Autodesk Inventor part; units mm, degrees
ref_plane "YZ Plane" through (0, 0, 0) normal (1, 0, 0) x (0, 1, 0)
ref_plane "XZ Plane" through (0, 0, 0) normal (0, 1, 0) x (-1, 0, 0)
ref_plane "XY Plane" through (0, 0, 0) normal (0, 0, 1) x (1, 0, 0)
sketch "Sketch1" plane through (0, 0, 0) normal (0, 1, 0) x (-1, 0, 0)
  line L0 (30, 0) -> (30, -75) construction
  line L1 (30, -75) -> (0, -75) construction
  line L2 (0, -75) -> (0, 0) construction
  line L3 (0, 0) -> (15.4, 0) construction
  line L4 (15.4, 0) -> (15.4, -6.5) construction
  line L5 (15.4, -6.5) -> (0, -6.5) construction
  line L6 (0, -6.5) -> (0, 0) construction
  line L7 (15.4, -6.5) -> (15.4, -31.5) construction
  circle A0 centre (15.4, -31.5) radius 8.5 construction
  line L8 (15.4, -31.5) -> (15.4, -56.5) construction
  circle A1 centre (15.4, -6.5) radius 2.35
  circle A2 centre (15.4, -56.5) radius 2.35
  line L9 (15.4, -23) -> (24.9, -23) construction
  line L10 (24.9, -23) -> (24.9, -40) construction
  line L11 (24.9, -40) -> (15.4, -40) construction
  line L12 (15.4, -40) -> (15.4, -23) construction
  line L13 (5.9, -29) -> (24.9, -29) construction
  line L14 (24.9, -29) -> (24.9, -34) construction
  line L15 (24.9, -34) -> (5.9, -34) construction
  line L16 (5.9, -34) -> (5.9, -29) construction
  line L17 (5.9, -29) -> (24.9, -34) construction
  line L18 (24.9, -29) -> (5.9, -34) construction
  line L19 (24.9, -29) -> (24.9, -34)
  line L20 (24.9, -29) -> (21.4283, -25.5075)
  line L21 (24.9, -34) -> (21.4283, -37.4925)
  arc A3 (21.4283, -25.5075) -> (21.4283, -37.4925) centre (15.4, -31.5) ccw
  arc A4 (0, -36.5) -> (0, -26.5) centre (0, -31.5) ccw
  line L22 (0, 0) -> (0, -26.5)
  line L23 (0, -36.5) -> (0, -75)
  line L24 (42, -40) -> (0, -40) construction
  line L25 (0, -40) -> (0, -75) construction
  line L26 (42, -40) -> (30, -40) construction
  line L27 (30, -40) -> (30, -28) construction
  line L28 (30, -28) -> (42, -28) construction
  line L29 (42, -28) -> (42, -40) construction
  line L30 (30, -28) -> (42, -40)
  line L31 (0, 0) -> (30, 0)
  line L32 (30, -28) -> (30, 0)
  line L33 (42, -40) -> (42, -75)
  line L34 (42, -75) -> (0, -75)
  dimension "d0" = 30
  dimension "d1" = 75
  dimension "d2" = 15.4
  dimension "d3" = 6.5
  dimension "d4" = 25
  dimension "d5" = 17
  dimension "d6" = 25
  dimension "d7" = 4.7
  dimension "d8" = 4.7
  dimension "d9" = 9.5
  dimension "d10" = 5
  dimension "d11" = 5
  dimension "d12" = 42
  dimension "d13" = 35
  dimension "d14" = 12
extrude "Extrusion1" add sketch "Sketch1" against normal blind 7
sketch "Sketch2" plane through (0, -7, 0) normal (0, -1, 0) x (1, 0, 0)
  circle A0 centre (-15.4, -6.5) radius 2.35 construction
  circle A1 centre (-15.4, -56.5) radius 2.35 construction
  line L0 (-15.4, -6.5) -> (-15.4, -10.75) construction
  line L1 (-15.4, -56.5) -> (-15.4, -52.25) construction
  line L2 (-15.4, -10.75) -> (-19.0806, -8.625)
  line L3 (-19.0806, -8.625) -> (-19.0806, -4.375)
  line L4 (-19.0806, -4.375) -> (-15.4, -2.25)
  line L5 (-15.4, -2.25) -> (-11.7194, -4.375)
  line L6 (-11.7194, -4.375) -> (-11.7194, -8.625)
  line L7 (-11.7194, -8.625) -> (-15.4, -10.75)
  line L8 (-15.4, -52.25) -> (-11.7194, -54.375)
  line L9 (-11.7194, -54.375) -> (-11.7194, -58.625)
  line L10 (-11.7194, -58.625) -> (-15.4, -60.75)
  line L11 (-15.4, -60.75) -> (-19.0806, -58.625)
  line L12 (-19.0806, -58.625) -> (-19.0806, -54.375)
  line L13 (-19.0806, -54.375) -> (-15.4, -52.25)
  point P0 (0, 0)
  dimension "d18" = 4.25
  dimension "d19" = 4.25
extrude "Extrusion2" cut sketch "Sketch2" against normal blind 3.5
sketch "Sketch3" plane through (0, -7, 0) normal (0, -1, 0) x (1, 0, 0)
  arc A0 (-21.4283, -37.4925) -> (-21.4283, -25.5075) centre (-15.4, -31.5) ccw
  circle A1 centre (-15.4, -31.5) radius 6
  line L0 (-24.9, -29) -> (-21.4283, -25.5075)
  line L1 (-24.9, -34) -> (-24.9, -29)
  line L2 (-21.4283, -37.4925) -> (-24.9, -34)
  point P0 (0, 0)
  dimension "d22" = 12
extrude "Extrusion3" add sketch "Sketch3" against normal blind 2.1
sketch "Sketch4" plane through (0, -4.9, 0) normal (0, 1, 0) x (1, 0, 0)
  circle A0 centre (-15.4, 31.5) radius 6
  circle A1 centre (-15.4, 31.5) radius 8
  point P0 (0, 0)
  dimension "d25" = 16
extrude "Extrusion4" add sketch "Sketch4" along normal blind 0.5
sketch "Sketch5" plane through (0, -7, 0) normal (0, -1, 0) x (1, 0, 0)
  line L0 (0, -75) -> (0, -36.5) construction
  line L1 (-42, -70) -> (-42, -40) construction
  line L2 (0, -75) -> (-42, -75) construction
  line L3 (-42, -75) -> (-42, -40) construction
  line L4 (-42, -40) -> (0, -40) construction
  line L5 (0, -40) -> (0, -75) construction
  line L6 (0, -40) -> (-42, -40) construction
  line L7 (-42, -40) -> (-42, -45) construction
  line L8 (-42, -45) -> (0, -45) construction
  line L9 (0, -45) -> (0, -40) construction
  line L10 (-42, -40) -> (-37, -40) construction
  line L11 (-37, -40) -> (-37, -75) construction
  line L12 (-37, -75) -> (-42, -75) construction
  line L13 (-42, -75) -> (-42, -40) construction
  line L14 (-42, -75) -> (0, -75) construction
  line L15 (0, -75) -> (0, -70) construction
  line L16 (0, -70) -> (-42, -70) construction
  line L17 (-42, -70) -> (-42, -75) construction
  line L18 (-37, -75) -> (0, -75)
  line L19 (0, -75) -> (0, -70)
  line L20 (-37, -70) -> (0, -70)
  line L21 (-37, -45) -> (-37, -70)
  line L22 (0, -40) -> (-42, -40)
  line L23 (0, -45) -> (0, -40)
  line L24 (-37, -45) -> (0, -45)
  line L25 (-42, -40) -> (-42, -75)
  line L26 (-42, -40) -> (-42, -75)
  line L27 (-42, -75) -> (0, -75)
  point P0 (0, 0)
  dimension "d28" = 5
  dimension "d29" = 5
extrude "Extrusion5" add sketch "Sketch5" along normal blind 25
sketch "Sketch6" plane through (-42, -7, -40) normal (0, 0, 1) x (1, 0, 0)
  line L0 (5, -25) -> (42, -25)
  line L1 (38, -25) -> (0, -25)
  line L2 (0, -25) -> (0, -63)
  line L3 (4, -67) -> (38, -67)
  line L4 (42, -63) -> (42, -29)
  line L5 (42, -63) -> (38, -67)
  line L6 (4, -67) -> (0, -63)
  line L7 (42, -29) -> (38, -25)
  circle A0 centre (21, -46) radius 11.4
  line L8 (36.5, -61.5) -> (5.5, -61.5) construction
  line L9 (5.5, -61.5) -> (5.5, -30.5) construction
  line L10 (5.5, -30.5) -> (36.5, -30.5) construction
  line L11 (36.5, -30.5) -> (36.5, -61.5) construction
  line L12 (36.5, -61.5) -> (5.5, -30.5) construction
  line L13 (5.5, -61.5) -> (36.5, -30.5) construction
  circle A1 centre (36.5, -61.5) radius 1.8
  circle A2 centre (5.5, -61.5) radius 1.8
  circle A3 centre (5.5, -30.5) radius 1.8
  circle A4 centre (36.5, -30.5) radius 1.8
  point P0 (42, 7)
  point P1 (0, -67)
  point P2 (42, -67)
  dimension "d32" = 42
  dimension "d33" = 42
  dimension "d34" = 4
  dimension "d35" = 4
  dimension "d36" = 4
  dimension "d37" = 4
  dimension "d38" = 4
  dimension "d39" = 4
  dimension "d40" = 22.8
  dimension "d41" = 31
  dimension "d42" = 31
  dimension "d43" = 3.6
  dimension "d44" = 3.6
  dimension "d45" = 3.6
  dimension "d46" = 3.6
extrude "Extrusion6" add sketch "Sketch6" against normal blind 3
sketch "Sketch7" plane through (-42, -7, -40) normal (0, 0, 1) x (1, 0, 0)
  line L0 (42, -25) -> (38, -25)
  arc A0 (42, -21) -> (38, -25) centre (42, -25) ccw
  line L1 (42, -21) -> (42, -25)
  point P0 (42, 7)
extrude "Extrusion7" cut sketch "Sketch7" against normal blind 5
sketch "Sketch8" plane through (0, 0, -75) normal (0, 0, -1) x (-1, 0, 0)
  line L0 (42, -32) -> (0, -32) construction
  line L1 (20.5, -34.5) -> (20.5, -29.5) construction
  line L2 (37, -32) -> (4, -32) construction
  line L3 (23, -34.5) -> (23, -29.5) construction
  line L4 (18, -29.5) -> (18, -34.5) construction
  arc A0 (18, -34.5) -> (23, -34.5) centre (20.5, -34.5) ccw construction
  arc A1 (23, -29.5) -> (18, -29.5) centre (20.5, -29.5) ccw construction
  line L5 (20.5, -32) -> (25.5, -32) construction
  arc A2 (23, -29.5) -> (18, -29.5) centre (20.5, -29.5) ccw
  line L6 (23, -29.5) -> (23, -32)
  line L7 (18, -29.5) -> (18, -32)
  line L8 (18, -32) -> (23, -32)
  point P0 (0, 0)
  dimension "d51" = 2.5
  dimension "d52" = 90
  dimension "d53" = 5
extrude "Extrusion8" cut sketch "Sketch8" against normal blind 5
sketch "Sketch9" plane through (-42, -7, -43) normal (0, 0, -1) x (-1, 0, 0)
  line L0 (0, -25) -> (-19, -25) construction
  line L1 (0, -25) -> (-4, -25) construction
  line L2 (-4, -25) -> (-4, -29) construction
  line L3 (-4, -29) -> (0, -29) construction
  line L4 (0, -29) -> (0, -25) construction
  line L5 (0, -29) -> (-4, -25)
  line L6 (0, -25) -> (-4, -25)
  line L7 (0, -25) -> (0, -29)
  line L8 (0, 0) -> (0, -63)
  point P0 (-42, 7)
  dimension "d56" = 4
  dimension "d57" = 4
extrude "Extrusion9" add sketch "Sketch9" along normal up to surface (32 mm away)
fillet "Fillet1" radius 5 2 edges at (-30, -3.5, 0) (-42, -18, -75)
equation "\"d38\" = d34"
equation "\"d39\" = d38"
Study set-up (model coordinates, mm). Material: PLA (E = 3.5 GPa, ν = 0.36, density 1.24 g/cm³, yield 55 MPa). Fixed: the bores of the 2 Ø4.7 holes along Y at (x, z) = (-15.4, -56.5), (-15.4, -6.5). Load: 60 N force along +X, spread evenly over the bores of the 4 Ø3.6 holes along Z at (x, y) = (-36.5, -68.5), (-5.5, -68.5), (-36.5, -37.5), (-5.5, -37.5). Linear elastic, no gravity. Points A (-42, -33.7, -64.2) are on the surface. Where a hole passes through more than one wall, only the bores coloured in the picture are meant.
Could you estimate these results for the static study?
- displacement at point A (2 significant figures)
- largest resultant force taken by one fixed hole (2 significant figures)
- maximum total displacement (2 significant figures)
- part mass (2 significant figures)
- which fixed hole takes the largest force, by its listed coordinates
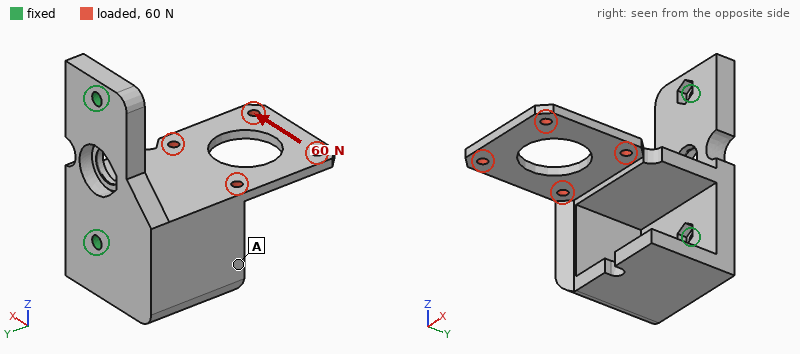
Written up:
0.50 mm
40 N
1.1 mm
43 g
(-15.4, -56.5)
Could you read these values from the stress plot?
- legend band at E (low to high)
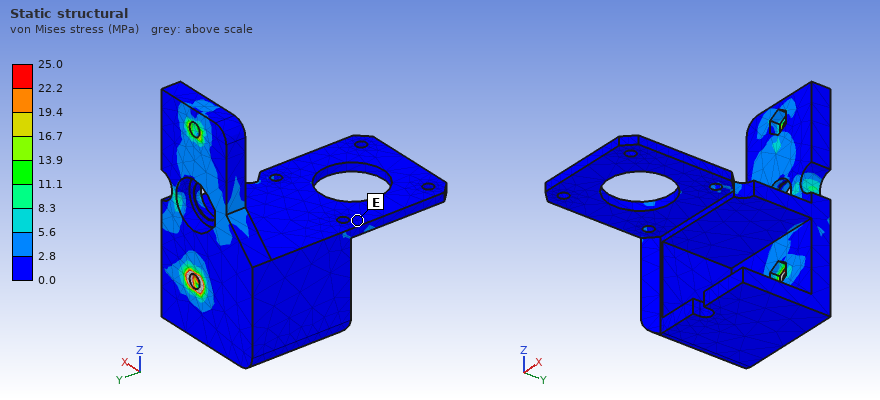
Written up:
0.0 to 2.8 MPa
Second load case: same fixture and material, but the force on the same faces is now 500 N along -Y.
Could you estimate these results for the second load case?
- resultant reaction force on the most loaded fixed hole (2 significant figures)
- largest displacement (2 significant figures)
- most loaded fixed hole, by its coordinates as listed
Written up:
450 N
1.3 mm
(-15.4, -56.5)
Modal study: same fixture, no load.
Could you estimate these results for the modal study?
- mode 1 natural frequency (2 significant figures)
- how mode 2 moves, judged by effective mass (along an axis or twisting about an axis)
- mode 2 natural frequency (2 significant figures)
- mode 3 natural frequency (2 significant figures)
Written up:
340 Hz
along X
460 Hz
840 Hz
